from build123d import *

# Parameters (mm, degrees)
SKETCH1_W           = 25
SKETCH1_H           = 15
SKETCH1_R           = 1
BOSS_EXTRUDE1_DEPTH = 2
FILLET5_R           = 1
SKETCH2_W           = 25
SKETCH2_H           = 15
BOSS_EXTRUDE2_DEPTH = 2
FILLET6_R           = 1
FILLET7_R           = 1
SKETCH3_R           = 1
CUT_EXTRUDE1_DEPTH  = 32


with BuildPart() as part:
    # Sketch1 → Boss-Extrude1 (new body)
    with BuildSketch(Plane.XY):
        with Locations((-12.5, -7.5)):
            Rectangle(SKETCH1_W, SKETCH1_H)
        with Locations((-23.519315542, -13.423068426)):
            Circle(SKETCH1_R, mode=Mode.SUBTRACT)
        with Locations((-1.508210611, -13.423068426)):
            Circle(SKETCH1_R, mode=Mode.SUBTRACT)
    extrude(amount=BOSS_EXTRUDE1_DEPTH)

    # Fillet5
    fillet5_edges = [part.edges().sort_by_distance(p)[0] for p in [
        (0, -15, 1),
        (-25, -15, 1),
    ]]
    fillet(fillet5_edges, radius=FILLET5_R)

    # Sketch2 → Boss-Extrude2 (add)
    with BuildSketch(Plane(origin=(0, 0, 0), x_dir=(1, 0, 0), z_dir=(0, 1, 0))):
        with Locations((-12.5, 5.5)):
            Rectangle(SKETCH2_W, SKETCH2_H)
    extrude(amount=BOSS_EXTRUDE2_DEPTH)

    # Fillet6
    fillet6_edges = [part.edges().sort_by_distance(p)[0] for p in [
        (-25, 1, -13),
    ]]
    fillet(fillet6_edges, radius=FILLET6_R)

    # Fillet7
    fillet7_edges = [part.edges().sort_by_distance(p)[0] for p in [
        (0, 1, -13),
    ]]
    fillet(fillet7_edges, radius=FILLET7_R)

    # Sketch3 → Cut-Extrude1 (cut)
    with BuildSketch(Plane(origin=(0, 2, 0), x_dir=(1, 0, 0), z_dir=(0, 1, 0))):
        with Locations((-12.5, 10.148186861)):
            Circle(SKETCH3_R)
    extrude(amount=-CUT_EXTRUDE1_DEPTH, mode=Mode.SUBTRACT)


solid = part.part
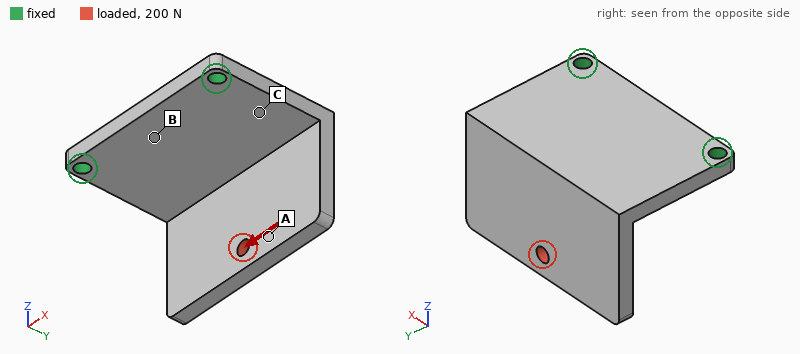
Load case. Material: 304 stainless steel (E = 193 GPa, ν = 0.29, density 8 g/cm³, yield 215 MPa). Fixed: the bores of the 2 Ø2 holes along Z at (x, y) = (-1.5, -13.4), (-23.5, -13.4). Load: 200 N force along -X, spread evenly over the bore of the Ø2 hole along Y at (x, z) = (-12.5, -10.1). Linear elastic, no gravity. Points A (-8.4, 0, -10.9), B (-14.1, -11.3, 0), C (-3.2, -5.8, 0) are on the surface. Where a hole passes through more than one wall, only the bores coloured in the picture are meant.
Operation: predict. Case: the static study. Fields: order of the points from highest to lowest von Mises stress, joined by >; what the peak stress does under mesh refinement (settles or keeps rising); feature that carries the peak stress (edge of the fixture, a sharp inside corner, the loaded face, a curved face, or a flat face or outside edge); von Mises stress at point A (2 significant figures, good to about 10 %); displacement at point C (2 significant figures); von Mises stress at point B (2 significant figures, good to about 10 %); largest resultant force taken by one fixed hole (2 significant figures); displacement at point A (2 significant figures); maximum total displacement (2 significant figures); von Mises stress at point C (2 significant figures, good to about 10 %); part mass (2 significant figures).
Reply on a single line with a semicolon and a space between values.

C > B > A; keeps rising; edge of the fixture; 18 MPa; 12 µm; 43 MPa; 190 N; 40 µm; 58 µm; 79 MPa; 12 g
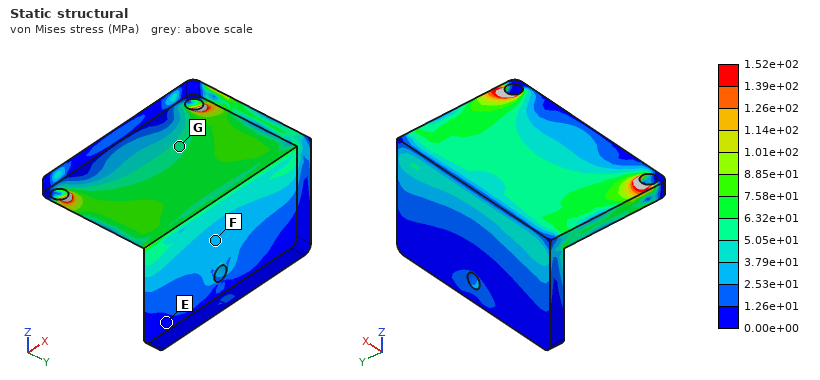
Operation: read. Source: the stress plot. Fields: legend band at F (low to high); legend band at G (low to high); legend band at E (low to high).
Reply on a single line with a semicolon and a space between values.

2.53e+01 to 3.79e+01 MPa; 5.05e+01 to 6.32e+01 MPa; 0.00e+00 to 1.26e+01 MPa
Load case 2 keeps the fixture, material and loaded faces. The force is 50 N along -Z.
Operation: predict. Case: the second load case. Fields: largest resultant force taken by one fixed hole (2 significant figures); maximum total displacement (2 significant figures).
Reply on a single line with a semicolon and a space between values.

25 N; 40 µm
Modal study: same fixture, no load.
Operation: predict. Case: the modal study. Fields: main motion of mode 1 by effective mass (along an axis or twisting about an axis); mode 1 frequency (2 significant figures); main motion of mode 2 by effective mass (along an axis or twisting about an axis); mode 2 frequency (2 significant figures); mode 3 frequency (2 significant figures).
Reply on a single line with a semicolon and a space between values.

along Z; 2200 Hz; along X; 4900 Hz; 6900 Hz
